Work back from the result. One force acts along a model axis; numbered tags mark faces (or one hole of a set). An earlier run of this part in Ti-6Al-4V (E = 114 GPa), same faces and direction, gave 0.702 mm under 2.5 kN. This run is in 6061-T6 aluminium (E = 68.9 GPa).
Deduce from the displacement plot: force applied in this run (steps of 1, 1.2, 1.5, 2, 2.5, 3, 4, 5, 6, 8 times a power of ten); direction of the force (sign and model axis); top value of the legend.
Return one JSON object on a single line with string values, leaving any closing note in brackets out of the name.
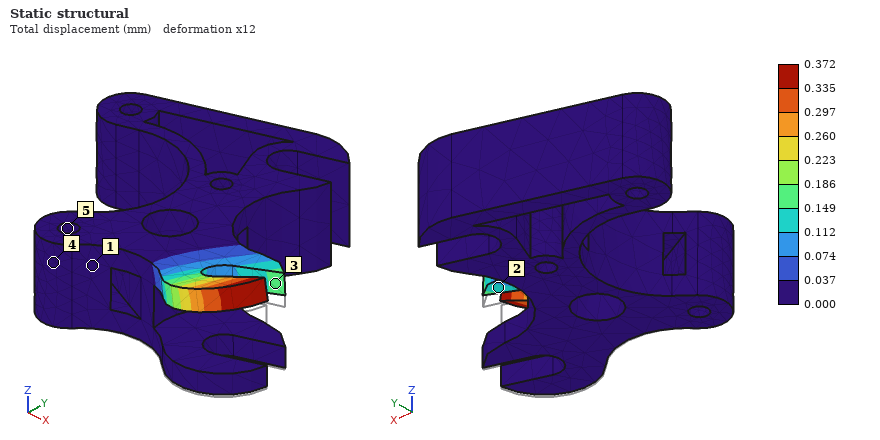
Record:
{"force applied in this run": "800 N", "direction of the force": "+Z", "top value of the legend": "0.372 mm"}
